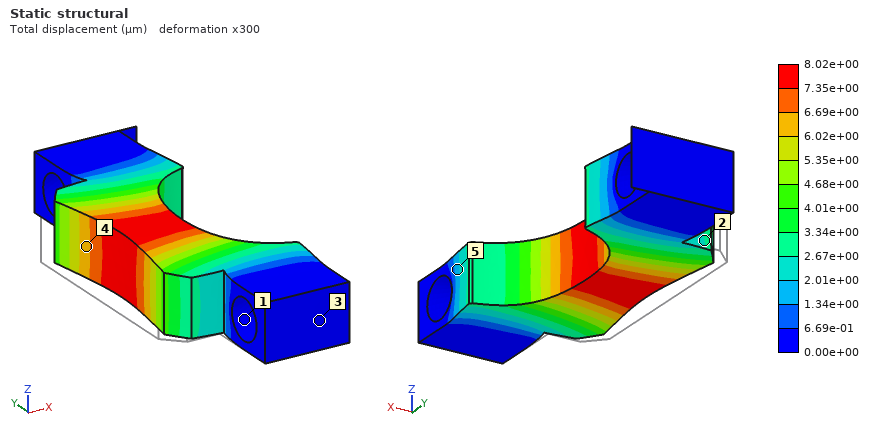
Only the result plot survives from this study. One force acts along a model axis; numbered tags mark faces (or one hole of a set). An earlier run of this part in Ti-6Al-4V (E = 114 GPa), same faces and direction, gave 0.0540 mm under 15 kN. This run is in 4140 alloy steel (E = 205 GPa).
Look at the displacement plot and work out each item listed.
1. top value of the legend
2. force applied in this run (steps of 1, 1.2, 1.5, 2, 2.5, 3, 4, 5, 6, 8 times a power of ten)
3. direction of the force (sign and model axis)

8.02e+00 µm
4 kN
+X
